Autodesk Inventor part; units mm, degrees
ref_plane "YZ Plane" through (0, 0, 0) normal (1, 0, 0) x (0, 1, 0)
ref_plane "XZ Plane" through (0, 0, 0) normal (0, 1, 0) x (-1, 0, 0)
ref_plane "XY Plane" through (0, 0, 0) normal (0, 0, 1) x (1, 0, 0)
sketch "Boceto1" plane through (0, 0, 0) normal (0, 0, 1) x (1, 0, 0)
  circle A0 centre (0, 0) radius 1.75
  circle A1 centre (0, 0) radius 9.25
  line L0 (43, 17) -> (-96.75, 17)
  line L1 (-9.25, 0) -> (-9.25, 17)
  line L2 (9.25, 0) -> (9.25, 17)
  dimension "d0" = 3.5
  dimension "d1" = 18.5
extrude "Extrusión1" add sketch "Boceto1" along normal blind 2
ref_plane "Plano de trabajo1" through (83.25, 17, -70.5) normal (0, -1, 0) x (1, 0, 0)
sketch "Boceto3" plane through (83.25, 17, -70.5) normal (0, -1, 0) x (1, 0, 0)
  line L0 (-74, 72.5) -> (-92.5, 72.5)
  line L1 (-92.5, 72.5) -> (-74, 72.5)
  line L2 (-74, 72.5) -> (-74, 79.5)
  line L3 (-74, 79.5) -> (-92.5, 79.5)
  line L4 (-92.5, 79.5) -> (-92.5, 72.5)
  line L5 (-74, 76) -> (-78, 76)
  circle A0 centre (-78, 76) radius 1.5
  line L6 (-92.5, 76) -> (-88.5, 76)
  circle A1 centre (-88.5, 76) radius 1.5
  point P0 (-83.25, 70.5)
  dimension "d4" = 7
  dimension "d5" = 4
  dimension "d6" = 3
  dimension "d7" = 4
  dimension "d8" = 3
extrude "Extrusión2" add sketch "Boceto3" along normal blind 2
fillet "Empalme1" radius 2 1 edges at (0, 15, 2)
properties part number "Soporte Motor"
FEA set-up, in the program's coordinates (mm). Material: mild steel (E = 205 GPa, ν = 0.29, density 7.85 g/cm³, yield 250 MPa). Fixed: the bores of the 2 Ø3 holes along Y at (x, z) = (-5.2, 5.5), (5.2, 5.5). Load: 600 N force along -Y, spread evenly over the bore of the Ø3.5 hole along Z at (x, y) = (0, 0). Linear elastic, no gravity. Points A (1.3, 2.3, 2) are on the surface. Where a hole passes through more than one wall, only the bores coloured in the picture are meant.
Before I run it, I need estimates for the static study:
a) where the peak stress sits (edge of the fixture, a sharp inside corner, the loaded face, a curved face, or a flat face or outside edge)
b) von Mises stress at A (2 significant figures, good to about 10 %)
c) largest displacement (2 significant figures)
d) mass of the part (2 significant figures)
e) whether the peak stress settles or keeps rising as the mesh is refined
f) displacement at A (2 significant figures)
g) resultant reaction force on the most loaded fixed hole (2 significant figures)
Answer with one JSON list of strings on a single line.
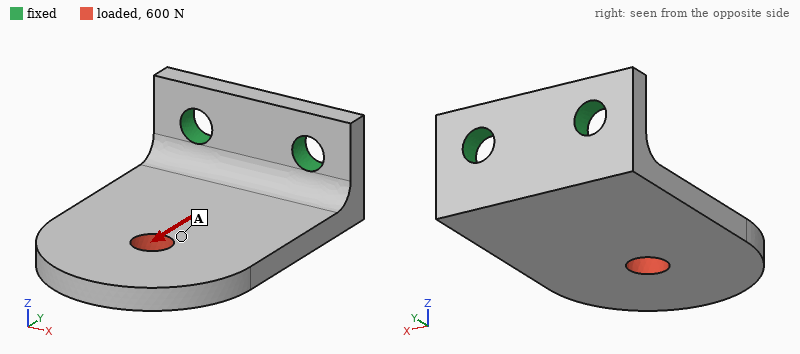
["edge of the fixture", "31 MPa", "40 µm", "8.8 g", "keeps rising", "22 µm", "300 N"]
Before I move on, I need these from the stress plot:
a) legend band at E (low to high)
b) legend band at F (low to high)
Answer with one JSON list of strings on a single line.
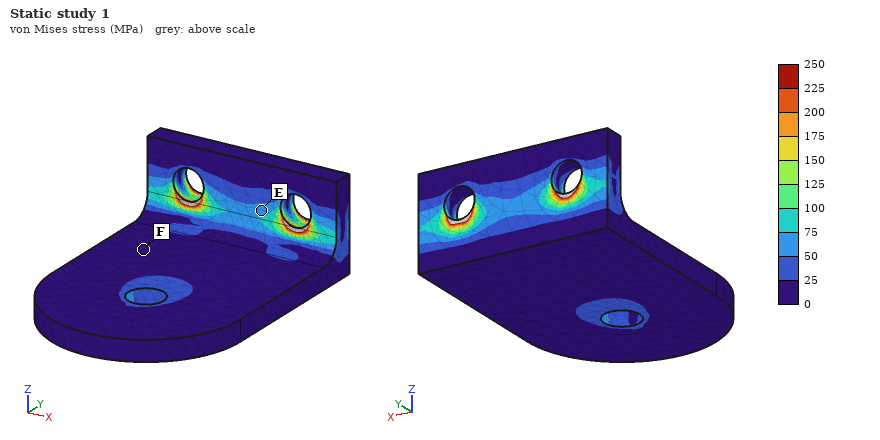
["50 to 75 MPa", "0 to 25 MPa"]
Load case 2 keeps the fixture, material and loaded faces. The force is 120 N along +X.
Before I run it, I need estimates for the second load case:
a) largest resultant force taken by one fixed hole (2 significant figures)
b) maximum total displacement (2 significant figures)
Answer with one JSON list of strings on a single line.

["170 N", "9.1 µm"]
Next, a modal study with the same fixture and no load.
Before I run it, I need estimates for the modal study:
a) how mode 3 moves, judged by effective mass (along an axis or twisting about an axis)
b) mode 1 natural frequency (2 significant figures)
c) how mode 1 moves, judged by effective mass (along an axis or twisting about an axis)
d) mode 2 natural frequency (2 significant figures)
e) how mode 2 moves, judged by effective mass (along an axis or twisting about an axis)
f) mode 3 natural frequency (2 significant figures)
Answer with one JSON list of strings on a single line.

["along X", "2800 Hz", "along Z", "8500 Hz", "along X", "12 kHz"]
